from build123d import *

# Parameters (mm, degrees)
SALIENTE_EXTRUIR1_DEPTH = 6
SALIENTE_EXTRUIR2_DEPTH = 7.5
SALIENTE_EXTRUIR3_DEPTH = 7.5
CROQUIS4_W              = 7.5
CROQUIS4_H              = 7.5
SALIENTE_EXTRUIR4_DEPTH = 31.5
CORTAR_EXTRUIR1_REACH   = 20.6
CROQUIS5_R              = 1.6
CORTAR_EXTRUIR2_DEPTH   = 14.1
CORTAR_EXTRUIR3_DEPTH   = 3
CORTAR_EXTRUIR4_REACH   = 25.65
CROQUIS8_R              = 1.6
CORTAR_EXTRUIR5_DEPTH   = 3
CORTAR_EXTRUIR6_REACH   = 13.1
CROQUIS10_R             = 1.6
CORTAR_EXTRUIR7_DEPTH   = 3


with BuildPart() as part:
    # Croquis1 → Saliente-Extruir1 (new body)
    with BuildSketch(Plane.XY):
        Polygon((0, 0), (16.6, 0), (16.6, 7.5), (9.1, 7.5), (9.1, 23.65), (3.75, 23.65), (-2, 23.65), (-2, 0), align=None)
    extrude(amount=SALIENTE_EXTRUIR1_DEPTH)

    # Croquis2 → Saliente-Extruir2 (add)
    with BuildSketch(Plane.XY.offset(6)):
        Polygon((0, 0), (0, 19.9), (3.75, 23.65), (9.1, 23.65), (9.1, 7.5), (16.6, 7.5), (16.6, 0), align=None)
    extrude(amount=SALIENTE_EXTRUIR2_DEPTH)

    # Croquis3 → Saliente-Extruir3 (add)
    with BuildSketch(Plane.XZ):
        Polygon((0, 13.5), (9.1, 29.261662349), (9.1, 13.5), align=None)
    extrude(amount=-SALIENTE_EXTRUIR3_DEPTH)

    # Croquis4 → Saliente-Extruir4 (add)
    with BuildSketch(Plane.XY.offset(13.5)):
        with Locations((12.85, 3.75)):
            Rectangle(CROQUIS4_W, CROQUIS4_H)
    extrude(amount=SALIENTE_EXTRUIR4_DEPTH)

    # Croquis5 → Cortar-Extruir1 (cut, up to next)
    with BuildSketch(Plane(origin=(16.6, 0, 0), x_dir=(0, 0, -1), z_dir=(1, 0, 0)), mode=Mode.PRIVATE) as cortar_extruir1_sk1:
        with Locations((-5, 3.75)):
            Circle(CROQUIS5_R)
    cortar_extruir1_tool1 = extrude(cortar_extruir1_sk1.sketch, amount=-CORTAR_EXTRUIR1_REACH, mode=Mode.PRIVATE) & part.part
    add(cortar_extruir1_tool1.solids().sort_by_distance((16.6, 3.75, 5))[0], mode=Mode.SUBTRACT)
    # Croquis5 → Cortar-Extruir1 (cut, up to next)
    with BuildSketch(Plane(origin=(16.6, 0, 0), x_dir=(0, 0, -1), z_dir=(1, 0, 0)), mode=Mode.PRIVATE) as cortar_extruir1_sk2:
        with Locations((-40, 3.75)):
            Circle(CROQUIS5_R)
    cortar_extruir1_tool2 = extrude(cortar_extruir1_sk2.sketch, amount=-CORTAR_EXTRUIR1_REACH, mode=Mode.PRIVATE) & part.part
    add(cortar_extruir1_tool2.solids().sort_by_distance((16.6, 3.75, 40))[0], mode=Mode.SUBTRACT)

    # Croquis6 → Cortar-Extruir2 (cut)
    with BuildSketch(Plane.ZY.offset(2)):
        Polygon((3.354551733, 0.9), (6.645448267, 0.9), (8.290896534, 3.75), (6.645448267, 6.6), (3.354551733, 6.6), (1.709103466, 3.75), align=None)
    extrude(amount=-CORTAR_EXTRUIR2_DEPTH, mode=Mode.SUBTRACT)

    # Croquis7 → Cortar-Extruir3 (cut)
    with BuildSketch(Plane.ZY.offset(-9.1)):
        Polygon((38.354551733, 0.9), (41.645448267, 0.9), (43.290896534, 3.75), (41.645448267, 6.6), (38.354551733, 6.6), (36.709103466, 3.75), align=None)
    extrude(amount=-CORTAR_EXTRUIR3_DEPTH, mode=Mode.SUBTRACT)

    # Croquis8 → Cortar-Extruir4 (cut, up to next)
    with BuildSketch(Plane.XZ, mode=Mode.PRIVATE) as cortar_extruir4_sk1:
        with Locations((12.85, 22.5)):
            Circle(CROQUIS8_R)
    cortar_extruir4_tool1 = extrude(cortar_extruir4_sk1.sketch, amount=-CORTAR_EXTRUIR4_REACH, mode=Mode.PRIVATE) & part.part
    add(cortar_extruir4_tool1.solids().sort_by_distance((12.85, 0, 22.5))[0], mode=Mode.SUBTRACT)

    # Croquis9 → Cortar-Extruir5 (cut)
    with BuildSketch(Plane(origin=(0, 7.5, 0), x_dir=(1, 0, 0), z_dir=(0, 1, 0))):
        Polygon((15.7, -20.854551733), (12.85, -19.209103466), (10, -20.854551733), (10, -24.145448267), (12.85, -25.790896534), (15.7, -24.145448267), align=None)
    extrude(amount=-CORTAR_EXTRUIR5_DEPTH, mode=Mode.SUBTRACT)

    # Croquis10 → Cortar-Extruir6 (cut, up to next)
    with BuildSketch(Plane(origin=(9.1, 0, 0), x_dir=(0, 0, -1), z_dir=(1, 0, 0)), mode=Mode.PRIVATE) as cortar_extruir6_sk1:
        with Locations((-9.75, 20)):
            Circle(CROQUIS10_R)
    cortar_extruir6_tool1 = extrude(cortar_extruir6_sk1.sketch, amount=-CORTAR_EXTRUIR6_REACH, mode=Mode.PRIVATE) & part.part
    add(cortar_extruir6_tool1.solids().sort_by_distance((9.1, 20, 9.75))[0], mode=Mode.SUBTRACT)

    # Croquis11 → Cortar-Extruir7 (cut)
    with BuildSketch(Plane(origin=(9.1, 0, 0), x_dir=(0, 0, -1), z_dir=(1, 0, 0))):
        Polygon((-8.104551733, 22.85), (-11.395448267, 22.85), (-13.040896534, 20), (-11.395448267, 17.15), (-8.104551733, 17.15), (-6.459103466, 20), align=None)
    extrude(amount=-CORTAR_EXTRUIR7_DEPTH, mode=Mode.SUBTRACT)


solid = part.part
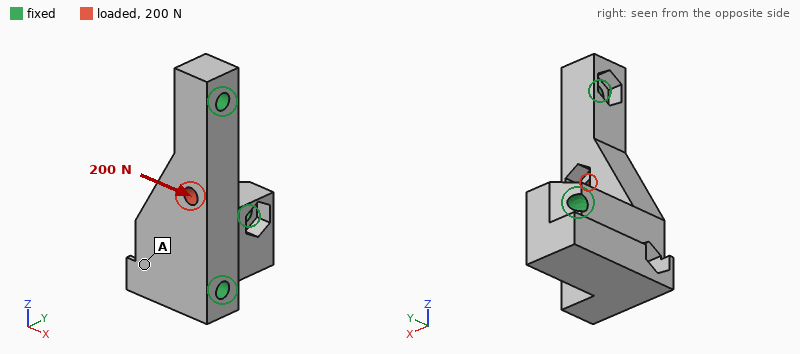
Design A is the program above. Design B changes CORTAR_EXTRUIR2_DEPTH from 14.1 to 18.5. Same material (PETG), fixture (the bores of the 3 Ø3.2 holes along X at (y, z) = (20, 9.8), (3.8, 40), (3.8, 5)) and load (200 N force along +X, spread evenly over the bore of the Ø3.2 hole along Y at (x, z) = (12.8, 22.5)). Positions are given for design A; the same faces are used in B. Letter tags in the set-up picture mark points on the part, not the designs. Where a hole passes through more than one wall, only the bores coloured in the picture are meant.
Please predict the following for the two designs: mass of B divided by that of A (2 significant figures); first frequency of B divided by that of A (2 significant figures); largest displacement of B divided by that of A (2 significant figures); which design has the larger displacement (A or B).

0.98
0.55
1.7
B
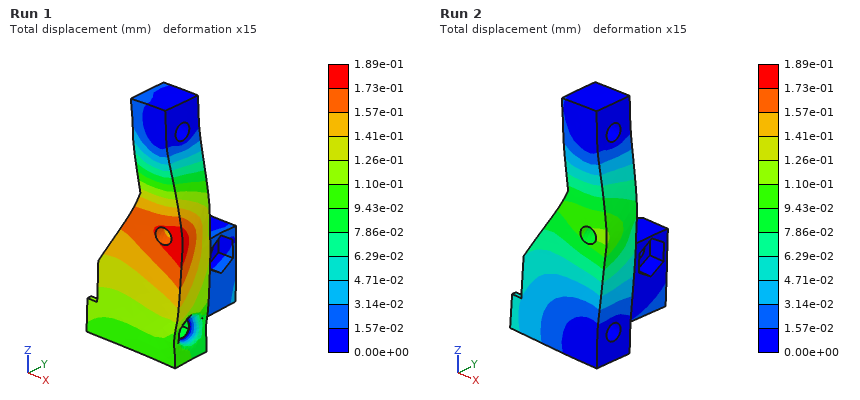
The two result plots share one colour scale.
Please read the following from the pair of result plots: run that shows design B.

Run 1
